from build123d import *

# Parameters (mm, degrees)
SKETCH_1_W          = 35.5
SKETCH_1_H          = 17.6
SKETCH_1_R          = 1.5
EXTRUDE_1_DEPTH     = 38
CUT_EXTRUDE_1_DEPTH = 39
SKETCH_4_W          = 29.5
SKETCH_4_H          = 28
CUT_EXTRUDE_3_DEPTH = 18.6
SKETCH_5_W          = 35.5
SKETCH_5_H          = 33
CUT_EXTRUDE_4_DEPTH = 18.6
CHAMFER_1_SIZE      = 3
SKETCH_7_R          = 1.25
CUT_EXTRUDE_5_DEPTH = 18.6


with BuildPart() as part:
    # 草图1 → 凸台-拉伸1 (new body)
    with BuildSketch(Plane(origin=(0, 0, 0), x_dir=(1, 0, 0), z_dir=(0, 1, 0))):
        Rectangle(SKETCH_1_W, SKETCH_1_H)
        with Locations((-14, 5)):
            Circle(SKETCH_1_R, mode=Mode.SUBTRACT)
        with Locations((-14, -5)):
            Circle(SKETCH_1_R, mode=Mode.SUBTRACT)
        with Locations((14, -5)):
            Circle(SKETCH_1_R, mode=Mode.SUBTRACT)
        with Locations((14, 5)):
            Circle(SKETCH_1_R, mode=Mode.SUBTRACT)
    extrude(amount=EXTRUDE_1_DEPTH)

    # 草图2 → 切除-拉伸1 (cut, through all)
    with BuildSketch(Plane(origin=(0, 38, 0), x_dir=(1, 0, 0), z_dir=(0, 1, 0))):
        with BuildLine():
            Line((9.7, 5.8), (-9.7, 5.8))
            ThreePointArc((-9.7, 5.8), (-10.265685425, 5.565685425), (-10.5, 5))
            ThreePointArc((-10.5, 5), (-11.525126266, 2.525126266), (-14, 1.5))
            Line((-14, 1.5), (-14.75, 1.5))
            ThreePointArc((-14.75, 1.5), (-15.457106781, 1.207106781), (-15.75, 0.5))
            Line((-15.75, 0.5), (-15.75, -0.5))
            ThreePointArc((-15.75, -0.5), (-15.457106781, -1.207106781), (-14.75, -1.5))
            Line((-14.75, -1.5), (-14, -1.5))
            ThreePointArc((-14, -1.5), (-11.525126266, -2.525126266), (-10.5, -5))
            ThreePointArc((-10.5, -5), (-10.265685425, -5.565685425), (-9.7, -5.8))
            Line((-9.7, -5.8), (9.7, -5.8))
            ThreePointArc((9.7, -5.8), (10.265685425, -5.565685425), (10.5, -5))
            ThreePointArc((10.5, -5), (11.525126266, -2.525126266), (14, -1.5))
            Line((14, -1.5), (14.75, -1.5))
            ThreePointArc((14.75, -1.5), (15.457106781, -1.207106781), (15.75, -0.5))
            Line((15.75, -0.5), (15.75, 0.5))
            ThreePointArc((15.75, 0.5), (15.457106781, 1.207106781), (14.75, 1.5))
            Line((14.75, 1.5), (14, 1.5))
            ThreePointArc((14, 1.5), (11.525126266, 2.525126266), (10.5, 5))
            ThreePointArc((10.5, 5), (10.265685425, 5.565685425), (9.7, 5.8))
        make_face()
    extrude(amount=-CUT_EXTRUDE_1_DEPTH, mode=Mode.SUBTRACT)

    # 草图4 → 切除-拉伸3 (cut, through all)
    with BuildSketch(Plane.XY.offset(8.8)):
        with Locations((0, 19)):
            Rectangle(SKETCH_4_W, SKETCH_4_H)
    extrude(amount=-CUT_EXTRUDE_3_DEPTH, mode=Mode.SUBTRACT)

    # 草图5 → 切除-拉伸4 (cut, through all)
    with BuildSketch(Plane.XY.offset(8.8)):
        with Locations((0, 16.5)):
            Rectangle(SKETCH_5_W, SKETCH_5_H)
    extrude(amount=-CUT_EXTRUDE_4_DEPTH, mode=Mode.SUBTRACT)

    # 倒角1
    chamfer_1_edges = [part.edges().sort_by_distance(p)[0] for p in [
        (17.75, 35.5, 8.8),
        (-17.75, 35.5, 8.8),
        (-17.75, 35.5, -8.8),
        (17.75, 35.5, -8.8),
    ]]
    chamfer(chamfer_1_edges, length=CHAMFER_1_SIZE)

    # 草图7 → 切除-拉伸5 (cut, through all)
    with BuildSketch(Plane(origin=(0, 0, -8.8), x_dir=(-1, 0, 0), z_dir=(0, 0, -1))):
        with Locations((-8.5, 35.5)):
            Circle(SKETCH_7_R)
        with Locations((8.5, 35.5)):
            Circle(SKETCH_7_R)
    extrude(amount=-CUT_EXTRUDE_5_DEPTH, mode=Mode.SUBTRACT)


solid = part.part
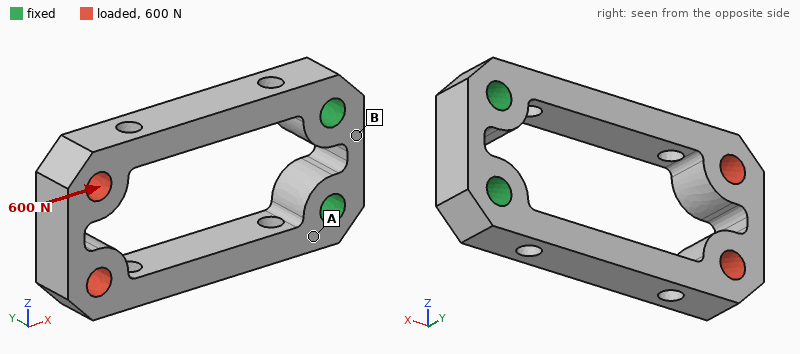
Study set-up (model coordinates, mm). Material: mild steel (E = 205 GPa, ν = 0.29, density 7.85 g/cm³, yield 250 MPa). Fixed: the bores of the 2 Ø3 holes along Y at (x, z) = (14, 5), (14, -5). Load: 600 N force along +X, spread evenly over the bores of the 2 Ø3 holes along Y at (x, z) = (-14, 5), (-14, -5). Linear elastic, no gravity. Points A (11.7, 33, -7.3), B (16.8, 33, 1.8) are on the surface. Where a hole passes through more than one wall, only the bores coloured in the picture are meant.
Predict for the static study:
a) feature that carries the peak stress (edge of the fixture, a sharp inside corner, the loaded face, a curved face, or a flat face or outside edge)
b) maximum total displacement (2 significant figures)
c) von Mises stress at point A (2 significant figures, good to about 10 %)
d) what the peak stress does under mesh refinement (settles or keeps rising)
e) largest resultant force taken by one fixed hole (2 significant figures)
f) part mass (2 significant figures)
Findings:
a sharp inside corner
9.6 µm
31 MPa
keeps rising
300 N
11 g
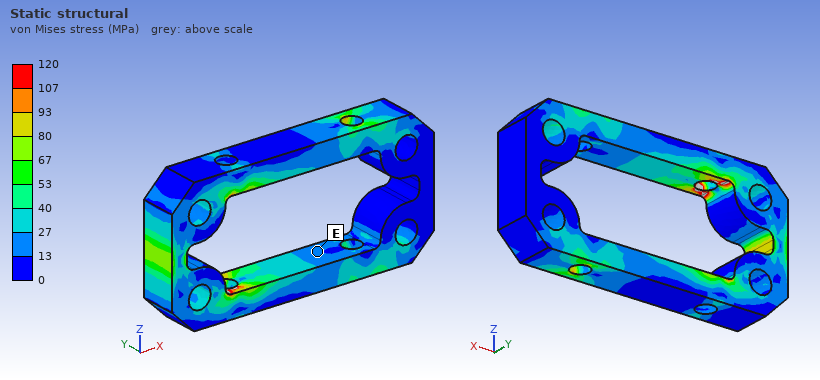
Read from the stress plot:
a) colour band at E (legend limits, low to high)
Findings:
13 to 27 MPa
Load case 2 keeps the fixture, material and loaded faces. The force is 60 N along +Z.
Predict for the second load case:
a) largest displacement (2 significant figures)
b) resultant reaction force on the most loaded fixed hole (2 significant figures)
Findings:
25 µm
71 N
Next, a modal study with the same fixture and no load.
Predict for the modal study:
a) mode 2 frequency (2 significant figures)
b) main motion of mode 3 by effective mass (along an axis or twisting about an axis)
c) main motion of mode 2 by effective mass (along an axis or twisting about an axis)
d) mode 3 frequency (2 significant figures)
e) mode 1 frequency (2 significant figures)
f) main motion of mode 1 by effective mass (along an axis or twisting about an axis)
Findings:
3600 Hz
twisting about X
along Z
7800 Hz
3300 Hz
along Y
